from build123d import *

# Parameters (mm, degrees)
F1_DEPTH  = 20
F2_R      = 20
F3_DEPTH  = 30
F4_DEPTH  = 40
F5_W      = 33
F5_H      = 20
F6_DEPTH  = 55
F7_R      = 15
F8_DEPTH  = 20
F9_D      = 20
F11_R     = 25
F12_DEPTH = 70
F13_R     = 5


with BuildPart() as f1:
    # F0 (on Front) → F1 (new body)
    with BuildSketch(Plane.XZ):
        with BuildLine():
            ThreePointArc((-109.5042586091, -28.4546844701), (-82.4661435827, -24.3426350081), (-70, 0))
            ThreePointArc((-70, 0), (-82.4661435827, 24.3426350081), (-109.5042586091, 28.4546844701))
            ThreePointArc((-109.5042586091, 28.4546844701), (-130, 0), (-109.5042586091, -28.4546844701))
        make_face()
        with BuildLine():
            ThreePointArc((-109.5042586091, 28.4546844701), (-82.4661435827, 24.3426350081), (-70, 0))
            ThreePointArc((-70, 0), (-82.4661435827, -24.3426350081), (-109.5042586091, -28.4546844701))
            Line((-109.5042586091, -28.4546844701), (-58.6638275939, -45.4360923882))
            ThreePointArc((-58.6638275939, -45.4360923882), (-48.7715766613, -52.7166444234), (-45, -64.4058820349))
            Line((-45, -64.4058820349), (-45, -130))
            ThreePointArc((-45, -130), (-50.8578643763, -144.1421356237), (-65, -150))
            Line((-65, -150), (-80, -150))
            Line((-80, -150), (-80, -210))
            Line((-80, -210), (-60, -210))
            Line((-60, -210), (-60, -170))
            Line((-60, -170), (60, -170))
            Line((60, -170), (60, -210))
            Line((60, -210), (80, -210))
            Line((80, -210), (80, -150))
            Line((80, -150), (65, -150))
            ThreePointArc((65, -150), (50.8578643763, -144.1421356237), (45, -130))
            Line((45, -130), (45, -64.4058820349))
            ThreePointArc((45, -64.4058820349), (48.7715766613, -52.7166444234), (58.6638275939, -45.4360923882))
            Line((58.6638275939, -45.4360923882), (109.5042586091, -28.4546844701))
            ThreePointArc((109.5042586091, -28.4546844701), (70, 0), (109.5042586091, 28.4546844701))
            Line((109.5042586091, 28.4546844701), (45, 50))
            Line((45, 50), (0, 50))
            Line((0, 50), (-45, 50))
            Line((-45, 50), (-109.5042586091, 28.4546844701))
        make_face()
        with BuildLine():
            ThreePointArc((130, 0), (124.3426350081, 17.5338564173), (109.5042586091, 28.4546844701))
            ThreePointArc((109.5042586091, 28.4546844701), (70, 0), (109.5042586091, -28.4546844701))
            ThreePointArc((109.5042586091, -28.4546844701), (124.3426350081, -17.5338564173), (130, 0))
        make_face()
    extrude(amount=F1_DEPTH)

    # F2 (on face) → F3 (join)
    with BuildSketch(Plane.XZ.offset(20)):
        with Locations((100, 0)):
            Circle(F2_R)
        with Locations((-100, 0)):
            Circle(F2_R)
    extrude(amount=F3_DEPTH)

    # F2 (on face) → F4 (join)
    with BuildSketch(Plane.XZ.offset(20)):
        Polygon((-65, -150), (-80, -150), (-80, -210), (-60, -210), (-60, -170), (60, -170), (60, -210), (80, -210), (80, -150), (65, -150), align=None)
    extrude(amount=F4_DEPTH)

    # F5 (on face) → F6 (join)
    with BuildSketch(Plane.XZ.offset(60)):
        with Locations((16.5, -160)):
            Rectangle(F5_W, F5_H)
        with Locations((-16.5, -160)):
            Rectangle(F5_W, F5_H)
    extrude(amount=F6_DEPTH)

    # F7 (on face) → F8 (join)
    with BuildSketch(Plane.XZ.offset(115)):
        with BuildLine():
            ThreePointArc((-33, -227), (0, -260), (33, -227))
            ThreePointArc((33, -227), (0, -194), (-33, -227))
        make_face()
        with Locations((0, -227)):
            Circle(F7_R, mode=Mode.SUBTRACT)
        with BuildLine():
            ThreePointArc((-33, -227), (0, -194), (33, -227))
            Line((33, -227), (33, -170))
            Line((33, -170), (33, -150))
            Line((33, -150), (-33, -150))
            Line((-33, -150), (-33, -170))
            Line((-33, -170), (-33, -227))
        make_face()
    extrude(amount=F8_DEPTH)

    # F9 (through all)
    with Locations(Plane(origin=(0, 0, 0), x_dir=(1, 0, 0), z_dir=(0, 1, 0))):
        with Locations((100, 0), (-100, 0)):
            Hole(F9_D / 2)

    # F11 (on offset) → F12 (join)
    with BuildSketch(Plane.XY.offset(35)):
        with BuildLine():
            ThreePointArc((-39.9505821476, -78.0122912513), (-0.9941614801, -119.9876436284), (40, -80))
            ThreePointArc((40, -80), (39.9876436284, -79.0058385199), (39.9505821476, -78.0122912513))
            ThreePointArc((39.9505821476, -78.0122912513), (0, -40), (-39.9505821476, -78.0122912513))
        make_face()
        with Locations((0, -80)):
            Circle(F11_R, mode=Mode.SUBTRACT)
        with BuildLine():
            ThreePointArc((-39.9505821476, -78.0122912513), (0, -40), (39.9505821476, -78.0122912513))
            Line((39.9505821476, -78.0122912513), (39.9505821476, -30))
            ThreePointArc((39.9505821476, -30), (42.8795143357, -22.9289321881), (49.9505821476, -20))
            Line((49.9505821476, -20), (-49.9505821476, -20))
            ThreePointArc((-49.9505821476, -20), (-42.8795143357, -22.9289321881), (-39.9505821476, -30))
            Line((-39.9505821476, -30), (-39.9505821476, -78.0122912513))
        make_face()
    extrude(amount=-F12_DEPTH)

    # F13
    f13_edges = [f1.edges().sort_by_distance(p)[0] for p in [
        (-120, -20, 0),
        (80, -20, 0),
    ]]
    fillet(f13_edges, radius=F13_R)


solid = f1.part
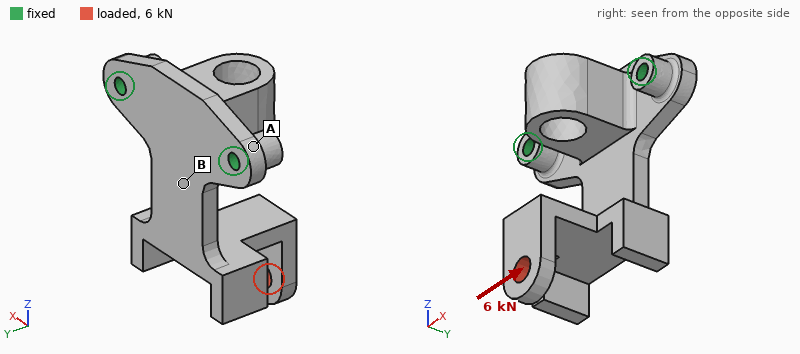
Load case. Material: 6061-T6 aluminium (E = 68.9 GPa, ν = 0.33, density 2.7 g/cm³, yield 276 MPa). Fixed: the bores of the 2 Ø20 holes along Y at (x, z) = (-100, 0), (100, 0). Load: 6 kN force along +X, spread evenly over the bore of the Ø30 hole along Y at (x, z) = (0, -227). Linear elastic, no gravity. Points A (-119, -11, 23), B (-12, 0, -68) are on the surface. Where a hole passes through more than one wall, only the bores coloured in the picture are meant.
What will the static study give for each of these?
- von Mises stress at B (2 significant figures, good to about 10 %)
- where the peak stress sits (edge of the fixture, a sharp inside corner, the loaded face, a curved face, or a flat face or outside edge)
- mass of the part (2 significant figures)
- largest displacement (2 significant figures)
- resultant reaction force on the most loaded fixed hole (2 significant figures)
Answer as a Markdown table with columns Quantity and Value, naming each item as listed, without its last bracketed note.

| Quantity | Value |
|---|---|
| von Mises stress at B | 87 MPa |
| where the peak stress sits | a curved face |
| mass of the part | 4.1 kg |
| largest displacement | 2.5 mm |
| resultant reaction force on the most loaded fixed hole | 9.4 kN |
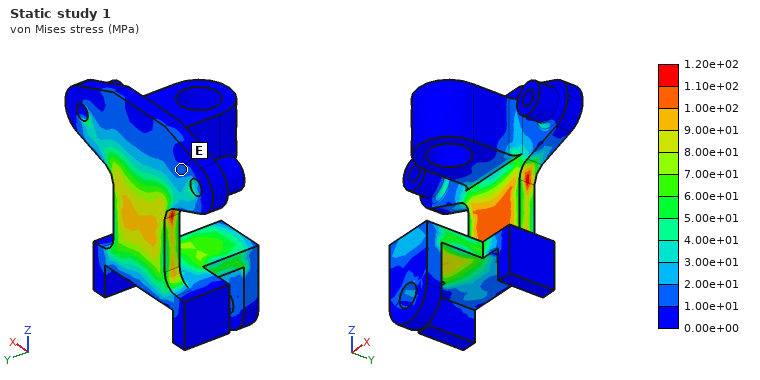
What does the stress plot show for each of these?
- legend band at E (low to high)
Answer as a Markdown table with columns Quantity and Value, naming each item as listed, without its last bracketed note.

| Quantity | Value |
|---|---|
| legend band at E | 1.00e+01 to 2.00e+01 MPa |
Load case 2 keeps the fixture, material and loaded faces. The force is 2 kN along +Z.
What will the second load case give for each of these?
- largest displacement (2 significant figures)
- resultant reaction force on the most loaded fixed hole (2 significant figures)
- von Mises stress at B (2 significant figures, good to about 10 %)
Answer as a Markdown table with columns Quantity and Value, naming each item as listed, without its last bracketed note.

| Quantity | Value |
|---|---|
| largest displacement | 2.1 mm |
| resultant reaction force on the most loaded fixed hole | 1.0 kN |
| von Mises stress at B | 34 MPa |
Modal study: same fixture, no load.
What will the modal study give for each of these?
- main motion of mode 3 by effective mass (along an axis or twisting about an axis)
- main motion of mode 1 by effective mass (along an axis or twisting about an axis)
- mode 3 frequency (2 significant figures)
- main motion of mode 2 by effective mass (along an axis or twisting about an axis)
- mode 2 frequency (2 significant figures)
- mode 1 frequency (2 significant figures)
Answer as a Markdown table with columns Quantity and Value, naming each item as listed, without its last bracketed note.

| Quantity | Value |
|---|---|
| main motion of mode 3 by effective mass | along Y |
| main motion of mode 1 by effective mass | along Y |
| mode 3 frequency | 610 Hz |
| main motion of mode 2 by effective mass | along X |
| mode 2 frequency | 380 Hz |
| mode 1 frequency | 180 Hz |
